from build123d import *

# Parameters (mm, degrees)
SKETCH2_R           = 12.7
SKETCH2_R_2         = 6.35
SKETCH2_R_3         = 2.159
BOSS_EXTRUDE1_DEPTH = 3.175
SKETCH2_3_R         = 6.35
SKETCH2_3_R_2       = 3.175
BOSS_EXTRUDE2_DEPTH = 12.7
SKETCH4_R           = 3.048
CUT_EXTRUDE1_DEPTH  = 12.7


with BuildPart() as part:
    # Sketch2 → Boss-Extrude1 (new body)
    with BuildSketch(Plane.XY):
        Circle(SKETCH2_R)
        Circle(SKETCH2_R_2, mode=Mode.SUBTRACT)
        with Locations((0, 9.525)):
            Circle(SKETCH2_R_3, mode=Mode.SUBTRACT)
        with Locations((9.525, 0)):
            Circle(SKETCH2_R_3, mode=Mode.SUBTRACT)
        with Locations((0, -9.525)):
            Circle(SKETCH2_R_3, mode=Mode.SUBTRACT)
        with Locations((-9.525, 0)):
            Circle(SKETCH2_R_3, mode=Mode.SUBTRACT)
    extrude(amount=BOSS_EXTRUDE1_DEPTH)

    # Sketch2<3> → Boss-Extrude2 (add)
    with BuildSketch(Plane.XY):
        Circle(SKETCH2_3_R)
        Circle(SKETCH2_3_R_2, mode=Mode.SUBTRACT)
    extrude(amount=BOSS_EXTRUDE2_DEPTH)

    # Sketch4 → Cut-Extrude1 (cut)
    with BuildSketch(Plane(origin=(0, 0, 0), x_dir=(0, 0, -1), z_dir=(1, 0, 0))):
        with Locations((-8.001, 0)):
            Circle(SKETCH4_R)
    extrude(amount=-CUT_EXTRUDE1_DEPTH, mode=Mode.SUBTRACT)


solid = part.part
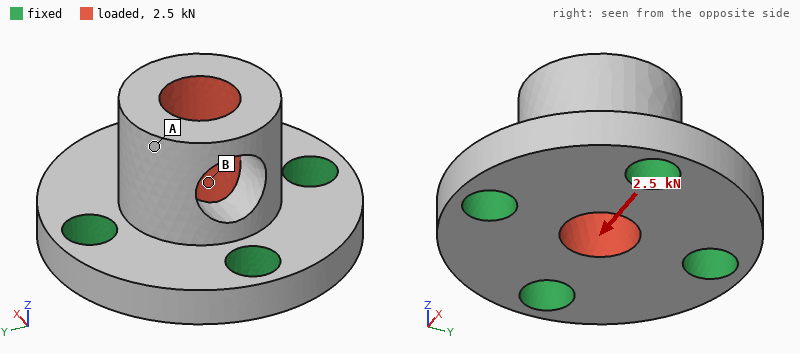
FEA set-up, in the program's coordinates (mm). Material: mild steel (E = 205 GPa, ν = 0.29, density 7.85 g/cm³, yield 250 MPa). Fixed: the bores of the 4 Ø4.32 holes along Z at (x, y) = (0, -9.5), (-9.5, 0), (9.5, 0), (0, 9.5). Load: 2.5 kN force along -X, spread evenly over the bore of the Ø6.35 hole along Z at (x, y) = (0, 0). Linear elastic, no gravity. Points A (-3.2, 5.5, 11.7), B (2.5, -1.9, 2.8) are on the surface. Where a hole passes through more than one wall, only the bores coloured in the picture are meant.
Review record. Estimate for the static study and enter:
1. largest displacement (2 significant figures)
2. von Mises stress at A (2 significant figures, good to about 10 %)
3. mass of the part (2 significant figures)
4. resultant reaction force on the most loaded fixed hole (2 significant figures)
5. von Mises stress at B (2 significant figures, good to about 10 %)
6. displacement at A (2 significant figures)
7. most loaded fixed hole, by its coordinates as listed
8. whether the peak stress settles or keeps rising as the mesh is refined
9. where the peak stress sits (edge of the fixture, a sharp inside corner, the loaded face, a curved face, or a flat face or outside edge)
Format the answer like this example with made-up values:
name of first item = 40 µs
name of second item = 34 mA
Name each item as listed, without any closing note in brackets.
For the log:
largest displacement = 7.0 µm
von Mises stress at A = 14 MPa
mass of the part = 17 g
resultant reaction force on the most loaded fixed hole = 1.2 kN
von Mises stress at B = 35 MPa
displacement at A = 5.3 µm
most loaded fixed hole, by its coordinates as listed = (9.5, 0)
whether the peak stress settles or keeps rising as the mesh is refined = keeps rising
where the peak stress sits = a sharp inside corner
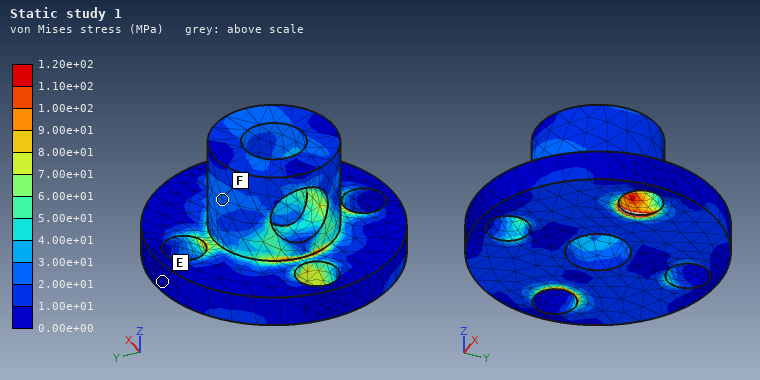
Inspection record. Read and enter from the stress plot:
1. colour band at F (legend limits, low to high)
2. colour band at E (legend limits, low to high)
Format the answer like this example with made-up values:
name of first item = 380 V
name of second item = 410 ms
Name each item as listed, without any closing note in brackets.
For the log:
colour band at F = 2.00e+01 to 3.00e+01 MPa
colour band at E = 0.00e+00 to 1.00e+01 MPa
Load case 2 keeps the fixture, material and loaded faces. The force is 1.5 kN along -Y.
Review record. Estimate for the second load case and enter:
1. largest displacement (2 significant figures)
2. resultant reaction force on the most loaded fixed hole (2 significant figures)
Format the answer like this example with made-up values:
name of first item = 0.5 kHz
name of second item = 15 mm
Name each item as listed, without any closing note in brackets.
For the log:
largest displacement = 4.7 µm
resultant reaction force on the most loaded fixed hole = 650 N
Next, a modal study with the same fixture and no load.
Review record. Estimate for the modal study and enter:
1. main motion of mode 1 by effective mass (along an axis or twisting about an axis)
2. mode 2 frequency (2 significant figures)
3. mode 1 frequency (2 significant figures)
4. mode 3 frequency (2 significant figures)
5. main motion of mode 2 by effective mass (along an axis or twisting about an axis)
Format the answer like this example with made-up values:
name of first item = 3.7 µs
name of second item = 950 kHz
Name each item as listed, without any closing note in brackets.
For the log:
main motion of mode 1 by effective mass = along Y
mode 2 frequency = 39 kHz
mode 1 frequency = 36 kHz
mode 3 frequency = 63 kHz
main motion of mode 2 by effective mass = along X
